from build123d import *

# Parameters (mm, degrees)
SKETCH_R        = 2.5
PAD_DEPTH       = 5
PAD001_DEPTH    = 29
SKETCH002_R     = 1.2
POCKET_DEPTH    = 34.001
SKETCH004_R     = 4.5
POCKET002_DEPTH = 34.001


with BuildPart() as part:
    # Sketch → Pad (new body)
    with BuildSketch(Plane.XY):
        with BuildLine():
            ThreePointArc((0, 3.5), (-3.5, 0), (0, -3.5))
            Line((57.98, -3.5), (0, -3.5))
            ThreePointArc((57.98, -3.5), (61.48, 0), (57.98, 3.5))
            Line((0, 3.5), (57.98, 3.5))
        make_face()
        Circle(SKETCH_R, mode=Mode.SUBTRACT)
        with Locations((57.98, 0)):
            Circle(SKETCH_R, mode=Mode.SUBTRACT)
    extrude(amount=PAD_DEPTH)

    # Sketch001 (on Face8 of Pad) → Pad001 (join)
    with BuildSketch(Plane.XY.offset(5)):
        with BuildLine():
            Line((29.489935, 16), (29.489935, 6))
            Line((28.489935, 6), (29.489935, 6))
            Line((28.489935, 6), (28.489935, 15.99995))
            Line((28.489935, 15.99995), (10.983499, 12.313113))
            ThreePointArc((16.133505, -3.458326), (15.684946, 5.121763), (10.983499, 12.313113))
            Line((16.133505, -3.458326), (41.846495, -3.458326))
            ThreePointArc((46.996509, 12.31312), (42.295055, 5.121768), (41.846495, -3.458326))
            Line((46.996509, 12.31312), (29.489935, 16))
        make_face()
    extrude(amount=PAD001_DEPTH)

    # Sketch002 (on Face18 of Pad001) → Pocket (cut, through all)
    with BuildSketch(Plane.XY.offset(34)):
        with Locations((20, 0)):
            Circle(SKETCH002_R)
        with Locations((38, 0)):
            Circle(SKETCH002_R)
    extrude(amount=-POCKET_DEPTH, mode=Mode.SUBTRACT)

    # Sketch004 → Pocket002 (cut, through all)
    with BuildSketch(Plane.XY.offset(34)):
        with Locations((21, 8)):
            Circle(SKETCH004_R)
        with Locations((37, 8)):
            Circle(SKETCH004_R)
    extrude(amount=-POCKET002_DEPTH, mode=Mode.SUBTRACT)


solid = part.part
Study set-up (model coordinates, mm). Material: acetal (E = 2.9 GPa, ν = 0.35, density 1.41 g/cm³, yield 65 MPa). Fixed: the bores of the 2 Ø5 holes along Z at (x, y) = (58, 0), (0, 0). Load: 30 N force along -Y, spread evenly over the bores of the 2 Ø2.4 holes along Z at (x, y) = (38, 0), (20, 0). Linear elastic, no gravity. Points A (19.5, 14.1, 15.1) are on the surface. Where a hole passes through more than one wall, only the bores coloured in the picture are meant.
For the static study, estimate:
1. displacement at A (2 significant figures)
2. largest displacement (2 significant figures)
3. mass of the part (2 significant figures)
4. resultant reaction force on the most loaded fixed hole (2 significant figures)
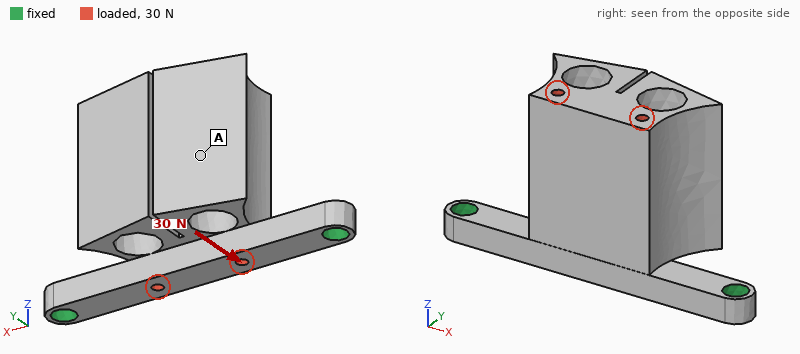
0.41 mm
0.75 mm
17 g
15 N
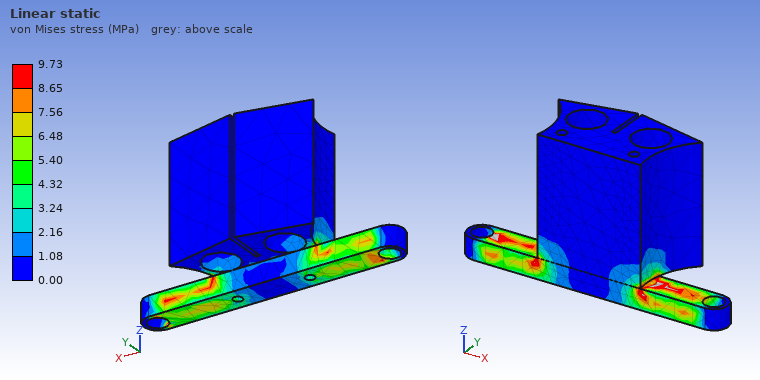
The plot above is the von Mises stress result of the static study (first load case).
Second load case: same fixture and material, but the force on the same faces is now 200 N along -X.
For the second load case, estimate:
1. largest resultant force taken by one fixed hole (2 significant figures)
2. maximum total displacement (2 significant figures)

120 N
0.36 mm
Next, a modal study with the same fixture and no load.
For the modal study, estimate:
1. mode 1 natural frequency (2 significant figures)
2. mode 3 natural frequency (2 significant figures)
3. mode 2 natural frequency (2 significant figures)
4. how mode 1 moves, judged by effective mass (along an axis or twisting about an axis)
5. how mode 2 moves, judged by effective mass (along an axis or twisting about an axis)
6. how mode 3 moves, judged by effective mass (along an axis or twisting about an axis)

290 Hz
1100 Hz
1000 Hz
along Y
along X
along Z
